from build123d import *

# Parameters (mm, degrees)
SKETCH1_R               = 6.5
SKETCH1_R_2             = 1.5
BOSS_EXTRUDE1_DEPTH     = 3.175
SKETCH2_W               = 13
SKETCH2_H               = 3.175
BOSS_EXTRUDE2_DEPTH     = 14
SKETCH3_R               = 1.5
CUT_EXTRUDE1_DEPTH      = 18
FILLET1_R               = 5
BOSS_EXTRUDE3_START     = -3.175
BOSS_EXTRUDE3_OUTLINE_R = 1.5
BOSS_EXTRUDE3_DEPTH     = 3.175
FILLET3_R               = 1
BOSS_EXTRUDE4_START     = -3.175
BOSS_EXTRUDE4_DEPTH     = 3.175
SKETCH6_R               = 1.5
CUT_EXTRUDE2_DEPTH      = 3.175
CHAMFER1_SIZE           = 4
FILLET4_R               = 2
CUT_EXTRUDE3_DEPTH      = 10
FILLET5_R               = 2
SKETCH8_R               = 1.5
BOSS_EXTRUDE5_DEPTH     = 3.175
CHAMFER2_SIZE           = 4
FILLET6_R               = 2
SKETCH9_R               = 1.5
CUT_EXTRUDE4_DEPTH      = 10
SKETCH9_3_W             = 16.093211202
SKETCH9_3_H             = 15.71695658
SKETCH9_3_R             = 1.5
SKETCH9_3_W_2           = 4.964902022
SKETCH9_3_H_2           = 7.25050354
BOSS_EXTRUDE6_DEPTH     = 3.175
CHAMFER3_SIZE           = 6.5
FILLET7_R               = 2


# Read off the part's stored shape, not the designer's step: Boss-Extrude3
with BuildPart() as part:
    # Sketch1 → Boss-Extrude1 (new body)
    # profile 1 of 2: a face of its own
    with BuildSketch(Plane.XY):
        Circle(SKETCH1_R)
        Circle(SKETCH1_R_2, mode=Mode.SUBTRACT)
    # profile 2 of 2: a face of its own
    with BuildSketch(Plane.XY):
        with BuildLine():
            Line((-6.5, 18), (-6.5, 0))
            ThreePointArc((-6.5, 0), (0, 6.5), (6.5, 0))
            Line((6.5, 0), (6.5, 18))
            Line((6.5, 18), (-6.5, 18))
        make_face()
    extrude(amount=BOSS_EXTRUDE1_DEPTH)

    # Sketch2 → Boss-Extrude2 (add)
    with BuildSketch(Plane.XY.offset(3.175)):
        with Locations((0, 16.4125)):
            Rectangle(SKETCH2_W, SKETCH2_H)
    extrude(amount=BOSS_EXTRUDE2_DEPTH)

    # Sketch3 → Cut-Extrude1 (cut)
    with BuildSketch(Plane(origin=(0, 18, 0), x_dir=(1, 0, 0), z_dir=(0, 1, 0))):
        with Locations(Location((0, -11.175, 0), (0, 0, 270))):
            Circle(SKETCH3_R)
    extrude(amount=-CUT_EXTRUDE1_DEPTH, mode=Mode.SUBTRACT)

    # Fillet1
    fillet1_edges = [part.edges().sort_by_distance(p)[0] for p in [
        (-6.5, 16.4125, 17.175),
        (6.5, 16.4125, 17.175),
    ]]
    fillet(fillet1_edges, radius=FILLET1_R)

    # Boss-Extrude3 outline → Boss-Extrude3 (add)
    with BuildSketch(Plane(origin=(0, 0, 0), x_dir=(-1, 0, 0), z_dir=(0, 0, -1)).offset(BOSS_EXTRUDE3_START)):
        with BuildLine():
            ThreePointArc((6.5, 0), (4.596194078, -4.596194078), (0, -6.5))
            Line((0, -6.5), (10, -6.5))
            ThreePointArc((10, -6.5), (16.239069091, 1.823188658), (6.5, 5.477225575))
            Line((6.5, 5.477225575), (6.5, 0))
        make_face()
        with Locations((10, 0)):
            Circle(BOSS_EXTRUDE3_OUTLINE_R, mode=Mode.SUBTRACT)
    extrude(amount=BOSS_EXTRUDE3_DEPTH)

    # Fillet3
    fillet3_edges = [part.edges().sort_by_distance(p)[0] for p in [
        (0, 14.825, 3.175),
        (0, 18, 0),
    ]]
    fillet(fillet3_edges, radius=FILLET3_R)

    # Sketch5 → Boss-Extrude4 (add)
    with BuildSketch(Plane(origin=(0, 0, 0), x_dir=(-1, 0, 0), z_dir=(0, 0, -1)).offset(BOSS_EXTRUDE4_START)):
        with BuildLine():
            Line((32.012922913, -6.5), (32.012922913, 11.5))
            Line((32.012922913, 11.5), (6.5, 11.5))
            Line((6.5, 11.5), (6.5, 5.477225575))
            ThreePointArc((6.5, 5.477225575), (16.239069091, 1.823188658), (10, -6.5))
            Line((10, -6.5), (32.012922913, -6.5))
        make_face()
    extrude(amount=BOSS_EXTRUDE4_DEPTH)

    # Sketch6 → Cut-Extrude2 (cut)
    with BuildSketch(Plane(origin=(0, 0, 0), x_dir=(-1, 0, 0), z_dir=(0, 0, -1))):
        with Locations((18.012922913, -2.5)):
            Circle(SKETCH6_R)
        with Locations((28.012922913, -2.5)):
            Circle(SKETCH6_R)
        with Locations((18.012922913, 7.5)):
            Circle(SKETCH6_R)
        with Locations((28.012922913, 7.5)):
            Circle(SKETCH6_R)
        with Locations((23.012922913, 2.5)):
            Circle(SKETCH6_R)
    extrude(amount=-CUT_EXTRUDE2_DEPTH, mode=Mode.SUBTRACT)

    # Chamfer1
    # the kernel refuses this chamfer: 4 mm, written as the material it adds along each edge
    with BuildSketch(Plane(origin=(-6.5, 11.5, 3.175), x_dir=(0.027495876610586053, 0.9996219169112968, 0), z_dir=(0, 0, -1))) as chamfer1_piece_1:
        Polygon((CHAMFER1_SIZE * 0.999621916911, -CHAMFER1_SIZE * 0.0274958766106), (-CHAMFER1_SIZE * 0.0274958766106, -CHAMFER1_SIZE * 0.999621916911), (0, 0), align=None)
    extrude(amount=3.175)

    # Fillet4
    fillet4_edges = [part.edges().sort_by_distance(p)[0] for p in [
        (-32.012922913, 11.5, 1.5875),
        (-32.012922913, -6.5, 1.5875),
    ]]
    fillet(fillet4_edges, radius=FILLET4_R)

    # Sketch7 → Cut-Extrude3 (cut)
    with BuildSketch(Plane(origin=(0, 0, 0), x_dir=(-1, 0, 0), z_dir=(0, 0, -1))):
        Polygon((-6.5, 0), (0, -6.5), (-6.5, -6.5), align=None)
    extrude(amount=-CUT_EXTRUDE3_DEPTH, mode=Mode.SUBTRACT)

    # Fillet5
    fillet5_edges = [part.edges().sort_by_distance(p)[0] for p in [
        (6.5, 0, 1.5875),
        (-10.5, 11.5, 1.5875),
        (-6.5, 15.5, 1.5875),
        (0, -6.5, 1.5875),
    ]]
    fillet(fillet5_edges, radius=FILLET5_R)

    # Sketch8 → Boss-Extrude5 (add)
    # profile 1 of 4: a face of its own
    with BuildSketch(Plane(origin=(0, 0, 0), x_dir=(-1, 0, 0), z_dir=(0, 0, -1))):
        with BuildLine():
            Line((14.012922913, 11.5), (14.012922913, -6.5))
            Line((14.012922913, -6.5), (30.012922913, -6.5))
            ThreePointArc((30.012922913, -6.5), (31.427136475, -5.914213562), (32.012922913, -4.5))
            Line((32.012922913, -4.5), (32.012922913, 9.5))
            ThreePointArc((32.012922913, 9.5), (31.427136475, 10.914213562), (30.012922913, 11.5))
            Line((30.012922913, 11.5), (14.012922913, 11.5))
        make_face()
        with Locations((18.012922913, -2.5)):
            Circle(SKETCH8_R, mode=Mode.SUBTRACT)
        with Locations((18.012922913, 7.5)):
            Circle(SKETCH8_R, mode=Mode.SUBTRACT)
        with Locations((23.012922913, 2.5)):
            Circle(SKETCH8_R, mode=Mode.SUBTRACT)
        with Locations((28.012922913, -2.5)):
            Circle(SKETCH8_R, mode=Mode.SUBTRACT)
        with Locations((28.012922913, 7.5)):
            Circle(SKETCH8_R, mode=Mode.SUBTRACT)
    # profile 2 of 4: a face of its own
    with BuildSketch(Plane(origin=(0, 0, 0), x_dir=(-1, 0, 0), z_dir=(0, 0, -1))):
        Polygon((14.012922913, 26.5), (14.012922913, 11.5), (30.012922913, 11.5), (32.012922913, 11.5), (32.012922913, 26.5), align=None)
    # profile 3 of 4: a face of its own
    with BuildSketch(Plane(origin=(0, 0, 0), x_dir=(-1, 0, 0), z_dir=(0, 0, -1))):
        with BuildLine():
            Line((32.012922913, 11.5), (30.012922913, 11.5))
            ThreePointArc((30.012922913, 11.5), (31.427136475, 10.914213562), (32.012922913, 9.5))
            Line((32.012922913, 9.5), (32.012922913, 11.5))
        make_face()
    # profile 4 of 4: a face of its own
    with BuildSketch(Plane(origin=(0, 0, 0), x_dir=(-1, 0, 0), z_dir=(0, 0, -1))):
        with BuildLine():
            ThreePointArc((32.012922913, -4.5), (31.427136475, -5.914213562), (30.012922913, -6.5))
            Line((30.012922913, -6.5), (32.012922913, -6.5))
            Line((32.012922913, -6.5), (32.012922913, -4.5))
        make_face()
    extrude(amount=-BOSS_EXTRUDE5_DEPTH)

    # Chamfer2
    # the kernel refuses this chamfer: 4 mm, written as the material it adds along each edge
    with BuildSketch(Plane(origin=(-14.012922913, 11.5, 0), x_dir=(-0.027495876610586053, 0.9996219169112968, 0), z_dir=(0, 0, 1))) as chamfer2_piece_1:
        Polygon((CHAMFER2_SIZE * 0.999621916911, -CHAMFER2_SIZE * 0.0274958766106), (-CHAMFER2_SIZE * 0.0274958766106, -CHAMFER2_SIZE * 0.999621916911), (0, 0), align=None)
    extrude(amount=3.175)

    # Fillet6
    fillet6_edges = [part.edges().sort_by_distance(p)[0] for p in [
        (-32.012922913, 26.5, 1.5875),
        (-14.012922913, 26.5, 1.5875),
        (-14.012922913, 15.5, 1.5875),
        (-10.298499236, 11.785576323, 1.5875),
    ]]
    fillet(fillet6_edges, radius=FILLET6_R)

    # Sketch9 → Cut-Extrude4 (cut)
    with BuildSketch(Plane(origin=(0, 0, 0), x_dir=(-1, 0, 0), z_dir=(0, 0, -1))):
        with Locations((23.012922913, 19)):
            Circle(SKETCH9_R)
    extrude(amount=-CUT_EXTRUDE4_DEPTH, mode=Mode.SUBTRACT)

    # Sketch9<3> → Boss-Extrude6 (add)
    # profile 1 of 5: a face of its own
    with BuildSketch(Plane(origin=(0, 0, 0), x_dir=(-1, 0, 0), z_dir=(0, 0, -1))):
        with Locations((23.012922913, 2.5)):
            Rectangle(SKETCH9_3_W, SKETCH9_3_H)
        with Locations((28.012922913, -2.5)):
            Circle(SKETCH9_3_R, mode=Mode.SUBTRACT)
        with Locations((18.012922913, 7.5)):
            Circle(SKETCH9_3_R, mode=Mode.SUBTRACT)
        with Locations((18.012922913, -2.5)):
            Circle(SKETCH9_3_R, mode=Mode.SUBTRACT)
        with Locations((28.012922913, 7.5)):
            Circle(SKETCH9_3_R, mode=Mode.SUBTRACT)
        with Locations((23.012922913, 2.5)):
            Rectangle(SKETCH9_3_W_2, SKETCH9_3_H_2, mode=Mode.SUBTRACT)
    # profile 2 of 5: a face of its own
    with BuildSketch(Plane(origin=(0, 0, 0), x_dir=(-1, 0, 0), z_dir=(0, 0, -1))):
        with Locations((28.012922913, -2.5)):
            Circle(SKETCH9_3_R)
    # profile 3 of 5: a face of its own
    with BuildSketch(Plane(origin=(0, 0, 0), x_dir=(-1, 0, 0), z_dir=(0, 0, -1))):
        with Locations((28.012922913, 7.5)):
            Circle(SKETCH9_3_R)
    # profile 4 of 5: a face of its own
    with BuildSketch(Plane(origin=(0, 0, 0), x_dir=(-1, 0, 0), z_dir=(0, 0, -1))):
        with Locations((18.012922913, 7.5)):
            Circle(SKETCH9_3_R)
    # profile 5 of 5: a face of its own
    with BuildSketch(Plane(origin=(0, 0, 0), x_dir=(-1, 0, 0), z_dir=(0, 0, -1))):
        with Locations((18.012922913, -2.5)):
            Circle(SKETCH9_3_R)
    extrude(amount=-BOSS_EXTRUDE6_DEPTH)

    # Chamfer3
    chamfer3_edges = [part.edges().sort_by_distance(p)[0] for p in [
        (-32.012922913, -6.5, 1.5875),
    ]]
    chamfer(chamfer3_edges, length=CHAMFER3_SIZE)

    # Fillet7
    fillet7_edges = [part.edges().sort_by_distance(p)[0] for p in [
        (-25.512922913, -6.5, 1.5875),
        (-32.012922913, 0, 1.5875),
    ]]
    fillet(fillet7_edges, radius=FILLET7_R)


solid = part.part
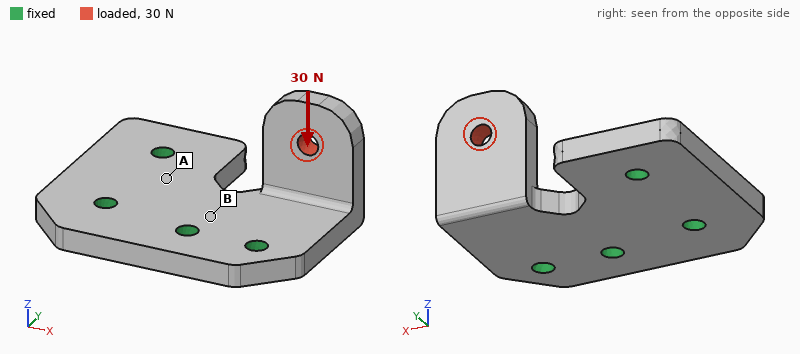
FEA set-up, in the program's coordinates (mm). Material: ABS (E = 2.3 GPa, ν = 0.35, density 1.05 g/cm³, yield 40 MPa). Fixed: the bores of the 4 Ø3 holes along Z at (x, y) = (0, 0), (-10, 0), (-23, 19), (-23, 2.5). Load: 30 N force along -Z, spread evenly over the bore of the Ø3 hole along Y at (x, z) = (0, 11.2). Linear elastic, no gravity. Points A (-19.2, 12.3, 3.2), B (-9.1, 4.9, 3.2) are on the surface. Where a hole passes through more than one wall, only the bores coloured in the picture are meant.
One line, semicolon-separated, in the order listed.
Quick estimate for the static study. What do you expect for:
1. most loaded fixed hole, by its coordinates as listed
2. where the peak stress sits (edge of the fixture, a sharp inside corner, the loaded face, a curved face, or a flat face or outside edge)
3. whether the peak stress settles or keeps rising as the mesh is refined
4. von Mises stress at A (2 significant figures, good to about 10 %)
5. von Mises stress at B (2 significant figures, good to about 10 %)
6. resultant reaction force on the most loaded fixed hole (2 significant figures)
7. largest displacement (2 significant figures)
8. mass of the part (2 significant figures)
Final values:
(0, 0); edge of the fixture; keeps rising; 2.3 MPa; 6.0 MPa; 24 N; 0.59 mm; 3.9 g
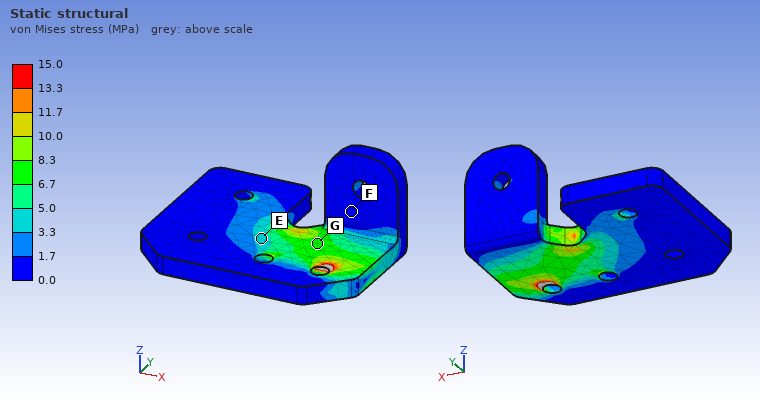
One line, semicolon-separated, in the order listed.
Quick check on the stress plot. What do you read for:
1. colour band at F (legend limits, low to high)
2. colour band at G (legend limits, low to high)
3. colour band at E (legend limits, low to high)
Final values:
0.0 to 1.7 MPa; 6.7 to 8.3 MPa; 3.3 to 5.0 MPa
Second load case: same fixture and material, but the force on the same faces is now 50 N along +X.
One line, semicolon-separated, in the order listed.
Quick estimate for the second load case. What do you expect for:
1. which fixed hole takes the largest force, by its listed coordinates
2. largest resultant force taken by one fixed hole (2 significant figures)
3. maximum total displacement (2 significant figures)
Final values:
(0, 0); 49 N; 0.62 mm
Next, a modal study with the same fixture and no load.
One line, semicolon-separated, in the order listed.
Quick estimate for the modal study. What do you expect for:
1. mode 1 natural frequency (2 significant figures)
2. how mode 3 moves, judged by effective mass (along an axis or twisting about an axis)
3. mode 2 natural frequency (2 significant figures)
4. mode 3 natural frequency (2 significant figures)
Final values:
1400 Hz; along Z; 2500 Hz; 3600 Hz
